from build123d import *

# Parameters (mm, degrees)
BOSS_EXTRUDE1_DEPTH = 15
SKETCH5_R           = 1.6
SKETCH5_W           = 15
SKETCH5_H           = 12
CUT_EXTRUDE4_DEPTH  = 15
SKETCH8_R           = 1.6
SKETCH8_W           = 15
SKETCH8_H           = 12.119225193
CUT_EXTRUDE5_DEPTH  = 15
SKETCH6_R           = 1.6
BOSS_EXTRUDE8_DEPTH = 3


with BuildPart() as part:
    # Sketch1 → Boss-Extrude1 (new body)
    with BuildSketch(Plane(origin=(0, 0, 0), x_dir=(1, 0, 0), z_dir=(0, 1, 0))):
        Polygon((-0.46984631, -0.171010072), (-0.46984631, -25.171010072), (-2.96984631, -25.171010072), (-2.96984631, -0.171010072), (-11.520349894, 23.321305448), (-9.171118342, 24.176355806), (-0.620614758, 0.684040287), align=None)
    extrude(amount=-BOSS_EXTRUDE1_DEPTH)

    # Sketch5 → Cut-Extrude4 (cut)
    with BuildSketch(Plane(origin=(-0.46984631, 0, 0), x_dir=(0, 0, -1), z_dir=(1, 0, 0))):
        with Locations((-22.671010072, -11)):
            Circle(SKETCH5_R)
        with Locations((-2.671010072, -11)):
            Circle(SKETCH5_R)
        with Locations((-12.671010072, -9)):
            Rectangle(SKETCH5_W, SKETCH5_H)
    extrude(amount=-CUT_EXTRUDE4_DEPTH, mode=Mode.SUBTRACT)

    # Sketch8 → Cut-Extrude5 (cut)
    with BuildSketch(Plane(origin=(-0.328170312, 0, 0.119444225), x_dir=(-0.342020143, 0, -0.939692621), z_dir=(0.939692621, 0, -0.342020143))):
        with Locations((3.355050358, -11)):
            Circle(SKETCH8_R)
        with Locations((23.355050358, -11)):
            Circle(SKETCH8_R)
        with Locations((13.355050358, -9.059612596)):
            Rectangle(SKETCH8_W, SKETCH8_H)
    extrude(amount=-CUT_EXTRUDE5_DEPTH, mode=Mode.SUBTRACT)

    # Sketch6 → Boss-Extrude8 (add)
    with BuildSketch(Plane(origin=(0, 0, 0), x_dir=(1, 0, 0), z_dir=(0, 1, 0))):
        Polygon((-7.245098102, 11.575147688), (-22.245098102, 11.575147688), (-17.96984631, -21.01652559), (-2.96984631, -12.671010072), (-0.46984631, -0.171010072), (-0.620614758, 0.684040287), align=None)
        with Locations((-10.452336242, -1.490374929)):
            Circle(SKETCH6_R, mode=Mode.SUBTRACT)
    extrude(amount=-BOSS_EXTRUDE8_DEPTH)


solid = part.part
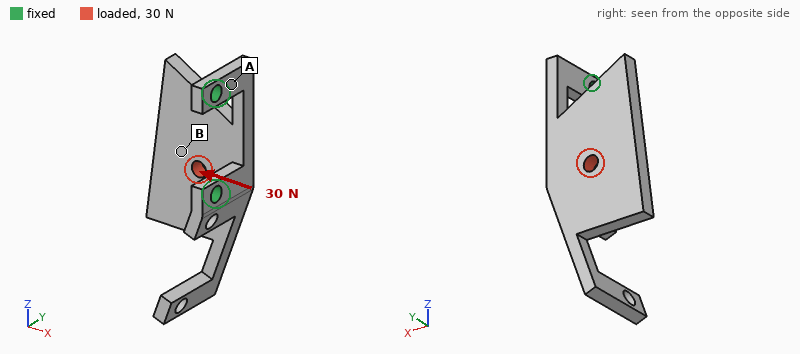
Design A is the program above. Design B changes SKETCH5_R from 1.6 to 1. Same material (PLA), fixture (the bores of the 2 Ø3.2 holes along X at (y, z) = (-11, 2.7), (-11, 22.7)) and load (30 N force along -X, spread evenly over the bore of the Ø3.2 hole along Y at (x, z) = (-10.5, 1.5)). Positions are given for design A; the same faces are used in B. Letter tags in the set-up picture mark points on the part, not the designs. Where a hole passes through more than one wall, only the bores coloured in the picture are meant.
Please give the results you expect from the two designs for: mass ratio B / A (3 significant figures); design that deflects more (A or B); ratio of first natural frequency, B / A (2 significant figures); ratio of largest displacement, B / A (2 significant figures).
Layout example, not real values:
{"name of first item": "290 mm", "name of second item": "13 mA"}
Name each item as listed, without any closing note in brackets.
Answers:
{"mass ratio B / A": "1.01", "design that deflects more": "B", "ratio of first natural frequency, B / A": "0.93", "ratio of largest displacement, B / A": "1.3"}
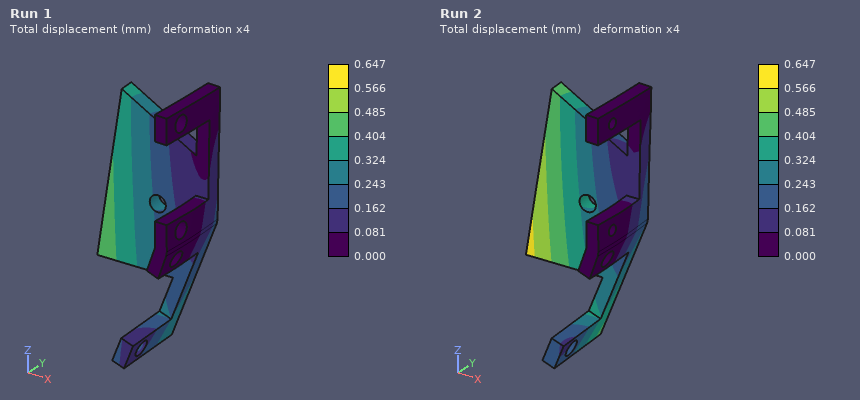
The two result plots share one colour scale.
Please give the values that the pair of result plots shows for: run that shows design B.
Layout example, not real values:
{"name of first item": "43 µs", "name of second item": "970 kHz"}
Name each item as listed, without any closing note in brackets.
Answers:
{"run that shows design B": "Run 2"}
